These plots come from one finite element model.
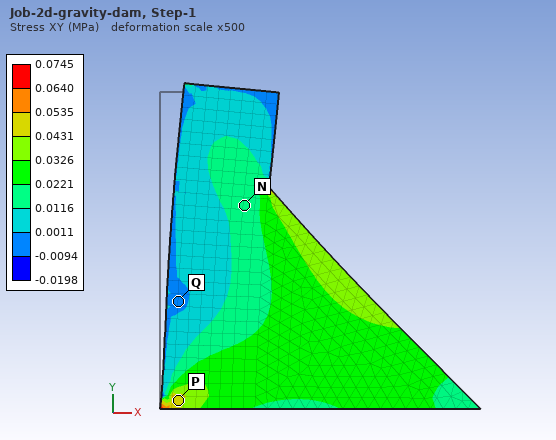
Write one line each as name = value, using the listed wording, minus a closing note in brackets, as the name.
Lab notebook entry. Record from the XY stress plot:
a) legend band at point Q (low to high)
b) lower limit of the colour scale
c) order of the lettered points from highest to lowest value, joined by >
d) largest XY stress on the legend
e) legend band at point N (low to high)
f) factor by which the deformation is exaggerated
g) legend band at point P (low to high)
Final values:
legend band at point Q = -0.0094 to 0.0011 MPa
lower limit of the colour scale = -0.0198 MPa
order of the lettered points from highest to lowest value, joined by > = P > N > Q
largest XY stress on the legend = 0.0745 MPa
legend band at point N = 0.0116 to 0.0221 MPa
factor by which the deformation is exaggerated = 500
legend band at point P = 0.0431 to 0.0535 MPa
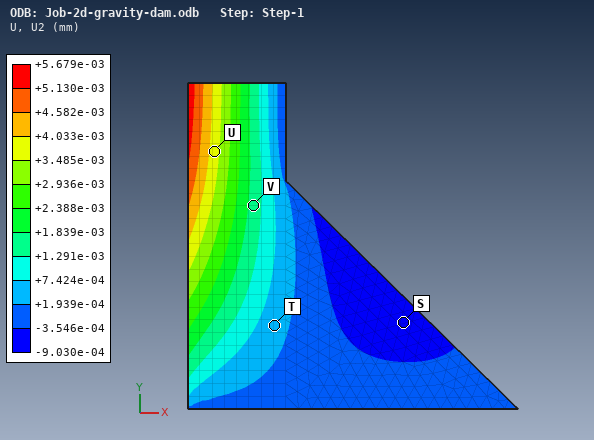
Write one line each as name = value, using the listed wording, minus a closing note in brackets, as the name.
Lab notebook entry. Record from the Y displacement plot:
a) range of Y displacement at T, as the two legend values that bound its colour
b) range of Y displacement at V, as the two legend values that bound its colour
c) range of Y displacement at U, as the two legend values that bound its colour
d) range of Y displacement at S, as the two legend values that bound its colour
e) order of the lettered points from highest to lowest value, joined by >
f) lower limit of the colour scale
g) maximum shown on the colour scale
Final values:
range of Y displacement at T, as the two legend values that bound its colour = +1.939e-04 to +7.424e-04 mm
range of Y displacement at V, as the two legend values that bound its colour = +1.291e-03 to +1.839e-03 mm
range of Y displacement at U, as the two legend values that bound its colour = +3.485e-03 to +4.033e-03 mm
range of Y displacement at S, as the two legend values that bound its colour = -9.030e-04 to -3.546e-04 mm
order of the lettered points from highest to lowest value, joined by > = U > V > T > S
lower limit of the colour scale = -9.030e-04 mm
maximum shown on the colour scale = +5.679e-03 mm
